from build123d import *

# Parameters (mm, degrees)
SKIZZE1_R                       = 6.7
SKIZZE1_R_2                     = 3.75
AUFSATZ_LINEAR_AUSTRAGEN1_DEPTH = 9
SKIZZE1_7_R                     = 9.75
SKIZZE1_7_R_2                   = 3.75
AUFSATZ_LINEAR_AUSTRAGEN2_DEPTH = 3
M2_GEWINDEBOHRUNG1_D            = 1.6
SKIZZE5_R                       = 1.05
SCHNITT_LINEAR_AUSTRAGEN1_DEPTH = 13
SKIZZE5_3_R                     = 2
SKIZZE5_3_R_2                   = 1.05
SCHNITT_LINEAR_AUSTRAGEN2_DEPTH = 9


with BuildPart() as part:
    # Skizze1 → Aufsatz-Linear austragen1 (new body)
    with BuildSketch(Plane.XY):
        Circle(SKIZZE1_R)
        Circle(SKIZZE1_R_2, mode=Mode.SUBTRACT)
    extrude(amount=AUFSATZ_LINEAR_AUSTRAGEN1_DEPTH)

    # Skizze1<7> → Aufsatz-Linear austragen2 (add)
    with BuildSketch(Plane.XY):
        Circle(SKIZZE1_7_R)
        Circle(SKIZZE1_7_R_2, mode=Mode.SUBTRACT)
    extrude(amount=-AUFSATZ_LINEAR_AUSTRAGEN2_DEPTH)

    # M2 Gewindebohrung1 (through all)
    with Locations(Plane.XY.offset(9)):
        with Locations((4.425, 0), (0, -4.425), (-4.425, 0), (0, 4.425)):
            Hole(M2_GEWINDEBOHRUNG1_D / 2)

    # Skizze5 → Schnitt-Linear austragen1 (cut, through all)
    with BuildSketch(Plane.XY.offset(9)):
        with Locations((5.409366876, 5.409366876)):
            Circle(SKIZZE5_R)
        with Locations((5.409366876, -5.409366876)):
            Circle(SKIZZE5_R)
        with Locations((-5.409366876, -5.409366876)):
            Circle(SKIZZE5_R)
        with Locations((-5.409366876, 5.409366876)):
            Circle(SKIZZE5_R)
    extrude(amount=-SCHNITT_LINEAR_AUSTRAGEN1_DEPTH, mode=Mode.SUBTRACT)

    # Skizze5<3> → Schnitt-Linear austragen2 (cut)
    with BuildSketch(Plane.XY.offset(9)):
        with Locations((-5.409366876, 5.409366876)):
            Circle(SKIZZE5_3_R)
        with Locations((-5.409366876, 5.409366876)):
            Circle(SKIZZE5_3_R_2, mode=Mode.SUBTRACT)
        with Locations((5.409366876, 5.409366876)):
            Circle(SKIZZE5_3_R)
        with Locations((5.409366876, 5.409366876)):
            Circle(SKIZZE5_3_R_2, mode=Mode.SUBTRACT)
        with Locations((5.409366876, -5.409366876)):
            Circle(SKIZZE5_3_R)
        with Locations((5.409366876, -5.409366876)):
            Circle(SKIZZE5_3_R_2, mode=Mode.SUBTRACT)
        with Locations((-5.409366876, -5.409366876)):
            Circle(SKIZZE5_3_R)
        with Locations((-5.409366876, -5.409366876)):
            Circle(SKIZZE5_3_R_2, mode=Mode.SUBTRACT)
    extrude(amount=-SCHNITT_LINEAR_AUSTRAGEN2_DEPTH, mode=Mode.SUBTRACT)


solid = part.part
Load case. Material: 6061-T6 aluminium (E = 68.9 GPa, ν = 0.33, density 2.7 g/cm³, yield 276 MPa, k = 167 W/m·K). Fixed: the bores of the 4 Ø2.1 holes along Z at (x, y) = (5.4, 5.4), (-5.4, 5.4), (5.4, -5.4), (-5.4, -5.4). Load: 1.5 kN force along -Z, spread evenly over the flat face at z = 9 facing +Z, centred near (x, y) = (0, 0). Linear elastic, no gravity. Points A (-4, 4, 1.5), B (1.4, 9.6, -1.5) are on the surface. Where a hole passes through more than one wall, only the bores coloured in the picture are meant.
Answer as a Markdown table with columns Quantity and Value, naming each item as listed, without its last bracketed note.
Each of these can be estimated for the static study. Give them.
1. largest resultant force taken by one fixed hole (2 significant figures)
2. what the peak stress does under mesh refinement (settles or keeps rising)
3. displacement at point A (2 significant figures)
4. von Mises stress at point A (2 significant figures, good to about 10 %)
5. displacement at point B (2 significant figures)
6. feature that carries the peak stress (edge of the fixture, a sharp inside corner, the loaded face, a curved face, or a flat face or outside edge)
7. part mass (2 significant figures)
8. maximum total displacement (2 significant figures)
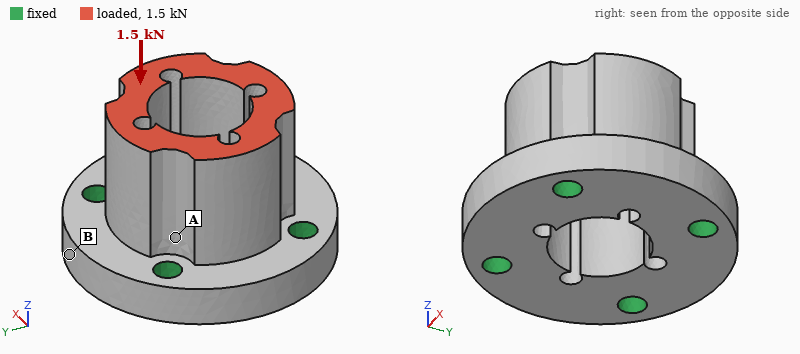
| Quantity | Value |
|---|---|
| largest resultant force taken by one fixed hole | 380 N |
| what the peak stress does under mesh refinement | keeps rising |
| displacement at point A | 2.7 µm |
| von Mises stress at point A | 27 MPa |
| displacement at point B | 1.4 µm |
| feature that carries the peak stress | edge of the fixture |
| part mass | 3.8 g |
| maximum total displacement | 4.9 µm |
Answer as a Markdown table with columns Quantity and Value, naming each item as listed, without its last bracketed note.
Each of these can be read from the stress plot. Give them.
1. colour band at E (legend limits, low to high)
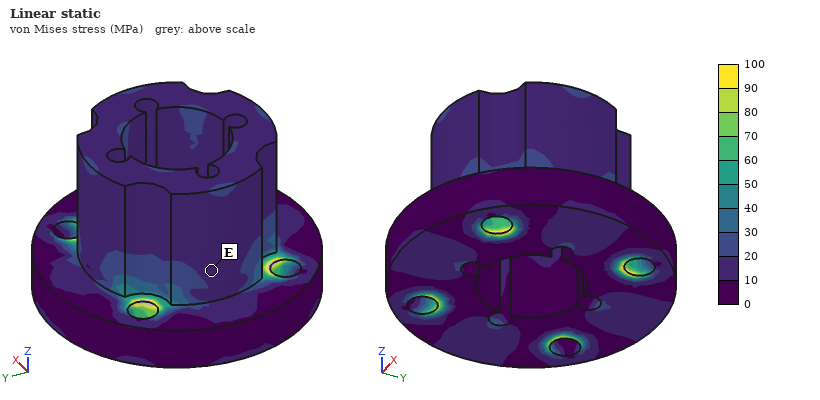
| Quantity | Value |
|---|---|
| colour band at E | 10 to 20 MPa |
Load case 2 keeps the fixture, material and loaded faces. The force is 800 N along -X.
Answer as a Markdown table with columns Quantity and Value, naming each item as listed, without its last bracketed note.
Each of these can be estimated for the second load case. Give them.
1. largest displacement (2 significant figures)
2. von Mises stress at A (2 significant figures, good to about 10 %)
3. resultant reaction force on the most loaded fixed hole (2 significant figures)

| Quantity | Value |
|---|---|
| largest displacement | 21 µm |
| von Mises stress at A | 42 MPa |
| resultant reaction force on the most loaded fixed hole | 430 N |
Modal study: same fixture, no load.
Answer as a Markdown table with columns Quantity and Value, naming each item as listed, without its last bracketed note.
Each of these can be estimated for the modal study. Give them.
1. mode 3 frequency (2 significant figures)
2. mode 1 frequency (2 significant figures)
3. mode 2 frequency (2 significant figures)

| Quantity | Value |
|---|---|
| mode 3 frequency | 42 kHz |
| mode 1 frequency | 39 kHz |
| mode 2 frequency | 39 kHz |
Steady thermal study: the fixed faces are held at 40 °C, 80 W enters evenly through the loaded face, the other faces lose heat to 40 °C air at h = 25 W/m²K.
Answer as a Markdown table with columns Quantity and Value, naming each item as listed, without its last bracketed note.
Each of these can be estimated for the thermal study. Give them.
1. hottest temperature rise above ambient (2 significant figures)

| Quantity | Value |
|---|---|
| hottest temperature rise above ambient | 69 K |
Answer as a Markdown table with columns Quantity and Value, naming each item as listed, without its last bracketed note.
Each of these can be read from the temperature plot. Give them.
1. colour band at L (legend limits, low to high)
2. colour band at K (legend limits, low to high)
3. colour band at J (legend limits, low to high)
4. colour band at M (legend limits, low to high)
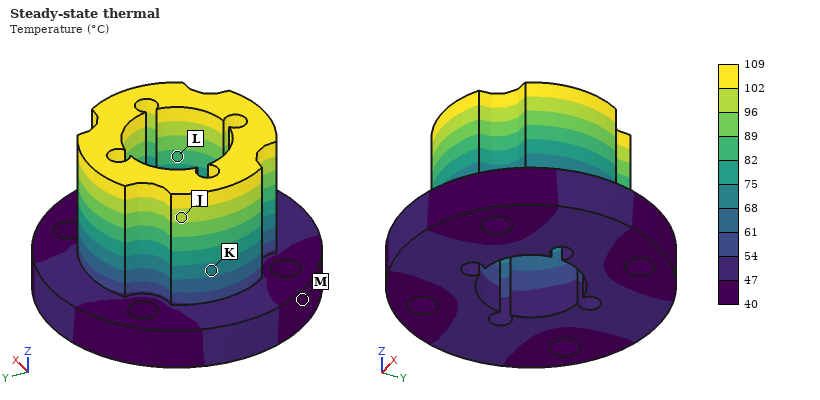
| Quantity | Value |
|---|---|
| colour band at L | 82 to 89 °C |
| colour band at K | 68 to 75 °C |
| colour band at J | 96 to 102 °C |
| colour band at M | 40 to 47 °C |
